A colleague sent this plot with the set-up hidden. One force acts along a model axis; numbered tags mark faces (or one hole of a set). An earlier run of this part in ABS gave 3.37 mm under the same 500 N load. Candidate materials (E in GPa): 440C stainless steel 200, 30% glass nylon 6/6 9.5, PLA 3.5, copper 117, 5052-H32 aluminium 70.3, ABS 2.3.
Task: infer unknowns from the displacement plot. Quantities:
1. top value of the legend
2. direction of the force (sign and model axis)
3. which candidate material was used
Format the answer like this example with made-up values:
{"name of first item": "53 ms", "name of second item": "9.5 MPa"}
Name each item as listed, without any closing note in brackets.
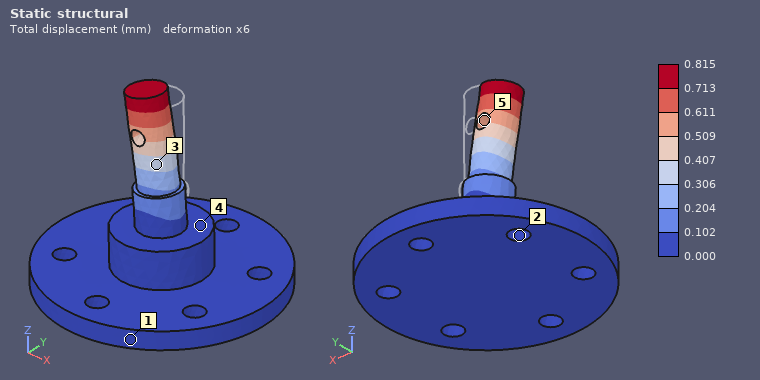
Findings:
{"top value of the legend": "0.815 mm", "direction of the force": "-X", "which candidate material was used": "30% glass nylon 6/6"}
